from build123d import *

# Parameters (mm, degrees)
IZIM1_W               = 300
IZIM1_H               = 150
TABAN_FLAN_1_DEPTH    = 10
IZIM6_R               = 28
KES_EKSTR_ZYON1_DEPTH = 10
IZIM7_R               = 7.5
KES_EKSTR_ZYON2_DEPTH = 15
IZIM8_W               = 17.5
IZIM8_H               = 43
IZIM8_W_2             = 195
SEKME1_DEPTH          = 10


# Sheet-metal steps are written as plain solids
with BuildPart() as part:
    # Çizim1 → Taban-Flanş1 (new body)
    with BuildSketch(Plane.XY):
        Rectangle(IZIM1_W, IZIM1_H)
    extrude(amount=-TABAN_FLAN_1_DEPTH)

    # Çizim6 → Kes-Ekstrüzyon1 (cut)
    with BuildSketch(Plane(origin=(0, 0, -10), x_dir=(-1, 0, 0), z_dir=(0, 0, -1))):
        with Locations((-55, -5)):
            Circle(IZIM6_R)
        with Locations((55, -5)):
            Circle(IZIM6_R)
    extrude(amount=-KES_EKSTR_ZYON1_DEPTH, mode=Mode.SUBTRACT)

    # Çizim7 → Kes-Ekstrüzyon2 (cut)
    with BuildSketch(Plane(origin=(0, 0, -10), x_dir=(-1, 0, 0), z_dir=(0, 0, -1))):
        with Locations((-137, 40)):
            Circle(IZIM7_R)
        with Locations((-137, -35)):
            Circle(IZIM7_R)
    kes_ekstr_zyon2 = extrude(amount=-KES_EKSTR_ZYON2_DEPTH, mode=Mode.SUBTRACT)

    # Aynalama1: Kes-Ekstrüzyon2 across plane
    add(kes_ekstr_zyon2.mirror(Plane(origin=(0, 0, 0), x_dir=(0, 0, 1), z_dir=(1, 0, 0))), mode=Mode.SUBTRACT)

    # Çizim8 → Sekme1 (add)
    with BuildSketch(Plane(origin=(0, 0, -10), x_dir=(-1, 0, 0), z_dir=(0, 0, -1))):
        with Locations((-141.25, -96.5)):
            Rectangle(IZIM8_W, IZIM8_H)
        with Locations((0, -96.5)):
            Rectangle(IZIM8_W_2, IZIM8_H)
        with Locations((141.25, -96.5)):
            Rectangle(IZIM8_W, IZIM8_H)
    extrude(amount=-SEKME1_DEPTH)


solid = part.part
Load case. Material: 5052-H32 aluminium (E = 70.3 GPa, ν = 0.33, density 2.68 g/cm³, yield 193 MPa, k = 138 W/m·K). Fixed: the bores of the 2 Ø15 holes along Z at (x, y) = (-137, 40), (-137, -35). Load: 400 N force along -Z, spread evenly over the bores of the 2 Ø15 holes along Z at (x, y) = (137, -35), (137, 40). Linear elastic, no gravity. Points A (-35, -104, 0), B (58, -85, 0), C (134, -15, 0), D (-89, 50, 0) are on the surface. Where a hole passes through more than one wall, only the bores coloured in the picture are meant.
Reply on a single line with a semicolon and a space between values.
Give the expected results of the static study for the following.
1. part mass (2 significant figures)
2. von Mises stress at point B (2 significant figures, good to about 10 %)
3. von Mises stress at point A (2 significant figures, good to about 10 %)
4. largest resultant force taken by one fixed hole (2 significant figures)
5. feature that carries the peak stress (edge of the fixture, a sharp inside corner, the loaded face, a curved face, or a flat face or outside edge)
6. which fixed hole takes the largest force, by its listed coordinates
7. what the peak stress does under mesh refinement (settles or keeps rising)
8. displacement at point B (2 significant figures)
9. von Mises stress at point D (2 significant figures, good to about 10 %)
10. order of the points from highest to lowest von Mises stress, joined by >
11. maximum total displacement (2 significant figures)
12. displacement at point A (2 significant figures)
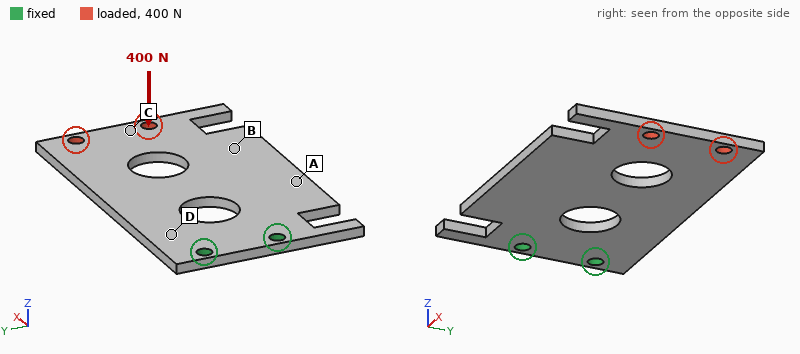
1.3 kg; 12 MPa; 22 MPa; 230 N; edge of the fixture; (-137, -35); keeps rising; 1.9 mm; 38 MPa; D > A > B > C; 3.5 mm; 0.62 mm
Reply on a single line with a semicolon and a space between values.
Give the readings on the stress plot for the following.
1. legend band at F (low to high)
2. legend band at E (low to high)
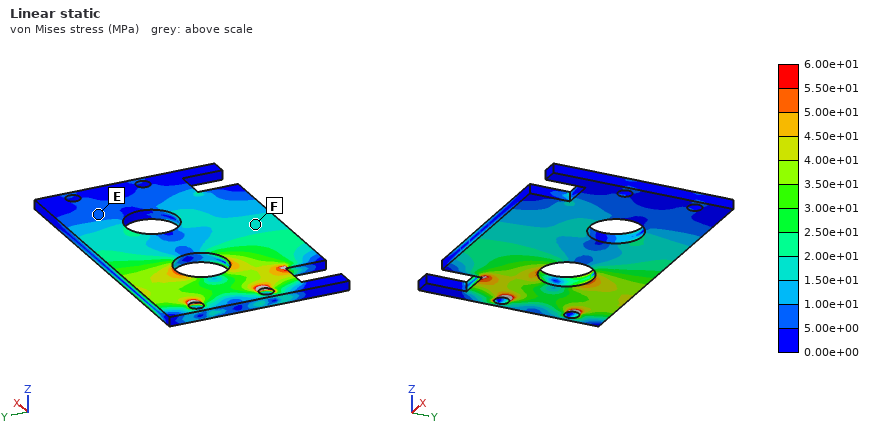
1.50e+01 to 2.00e+01 MPa; 5.00e+00 to 1.00e+01 MPa
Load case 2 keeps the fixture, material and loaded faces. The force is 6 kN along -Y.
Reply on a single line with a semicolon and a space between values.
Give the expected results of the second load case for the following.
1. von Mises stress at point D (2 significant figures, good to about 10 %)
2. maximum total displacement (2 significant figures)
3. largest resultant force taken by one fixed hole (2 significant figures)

30 MPa; 0.44 mm; 19 kN
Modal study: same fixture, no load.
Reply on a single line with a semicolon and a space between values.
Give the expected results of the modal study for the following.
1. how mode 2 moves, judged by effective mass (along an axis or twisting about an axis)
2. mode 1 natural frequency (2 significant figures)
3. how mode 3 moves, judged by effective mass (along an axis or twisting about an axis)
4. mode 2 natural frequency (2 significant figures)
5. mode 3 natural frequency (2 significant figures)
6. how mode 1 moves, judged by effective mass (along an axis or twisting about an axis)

twisting about X; 94 Hz; along Z; 290 Hz; 580 Hz; along Z
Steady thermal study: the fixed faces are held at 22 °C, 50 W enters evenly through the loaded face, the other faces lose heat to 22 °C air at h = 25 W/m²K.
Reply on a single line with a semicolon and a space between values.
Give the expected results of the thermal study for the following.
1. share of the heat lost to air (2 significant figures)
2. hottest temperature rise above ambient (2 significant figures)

75 %; 39 K
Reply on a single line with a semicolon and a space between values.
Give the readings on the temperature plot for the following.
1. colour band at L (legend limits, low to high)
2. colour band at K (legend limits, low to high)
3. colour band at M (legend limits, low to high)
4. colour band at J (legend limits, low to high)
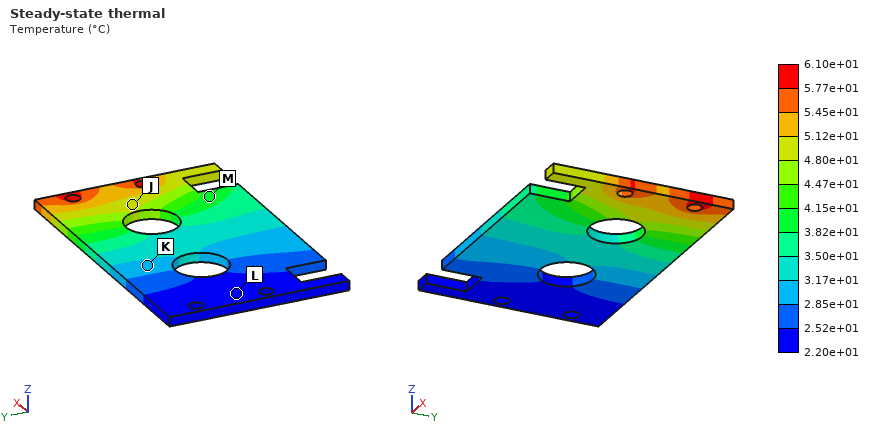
2.20e+01 to 2.52e+01 °C; 2.85e+01 to 3.17e+01 °C; 3.82e+01 to 4.15e+01 °C; 4.80e+01 to 5.12e+01 °C
